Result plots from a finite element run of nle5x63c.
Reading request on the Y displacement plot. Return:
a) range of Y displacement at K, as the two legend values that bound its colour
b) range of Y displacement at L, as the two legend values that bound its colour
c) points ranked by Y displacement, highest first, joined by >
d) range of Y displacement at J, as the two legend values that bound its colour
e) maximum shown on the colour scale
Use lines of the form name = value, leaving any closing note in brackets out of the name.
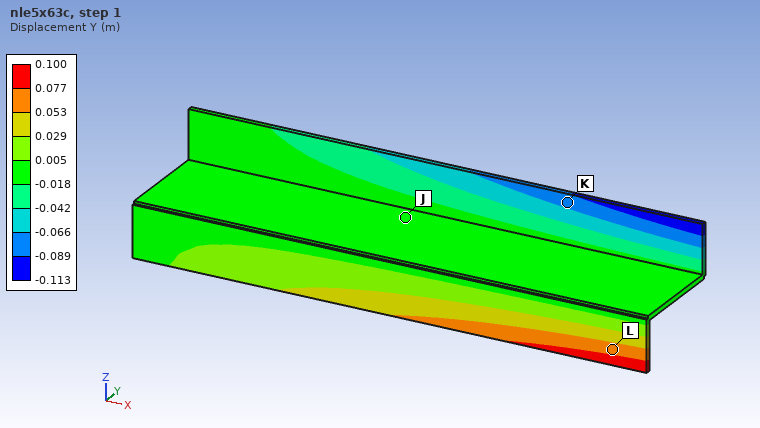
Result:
range of Y displacement at K, as the two legend values that bound its colour = -0.089 to -0.066 m
range of Y displacement at L, as the two legend values that bound its colour = 0.053 to 0.077 m
points ranked by Y displacement, highest first, joined by > = L > J > K
range of Y displacement at J, as the two legend values that bound its colour = -0.018 to 0.005 m
maximum shown on the colour scale = 0.100 m
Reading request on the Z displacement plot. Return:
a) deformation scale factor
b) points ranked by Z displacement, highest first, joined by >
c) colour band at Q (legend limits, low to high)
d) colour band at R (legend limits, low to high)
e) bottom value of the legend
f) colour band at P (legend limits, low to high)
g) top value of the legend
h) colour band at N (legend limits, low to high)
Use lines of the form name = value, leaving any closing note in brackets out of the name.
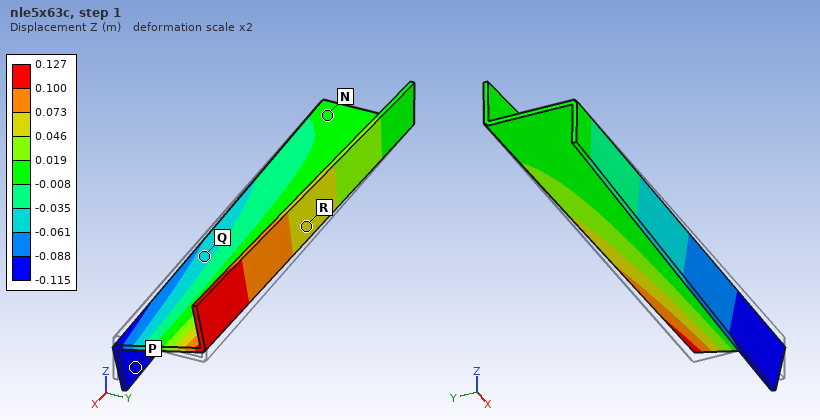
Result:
deformation scale factor = 2
points ranked by Z displacement, highest first, joined by > = R > N > Q > P
colour band at Q = -0.061 to -0.035 m
colour band at R = 0.046 to 0.073 m
bottom value of the legend = -0.115 m
colour band at P = -0.115 to -0.088 m
top value of the legend = 0.127 m
colour band at N = -0.008 to 0.019 m
